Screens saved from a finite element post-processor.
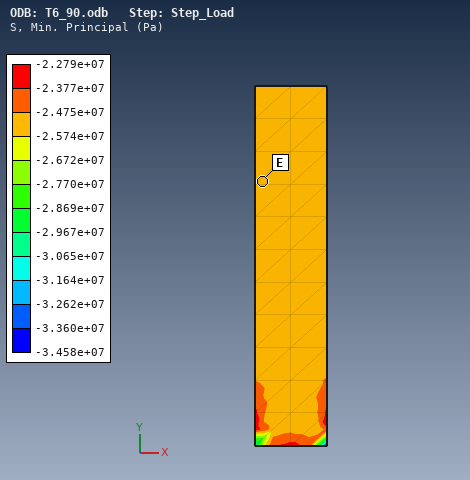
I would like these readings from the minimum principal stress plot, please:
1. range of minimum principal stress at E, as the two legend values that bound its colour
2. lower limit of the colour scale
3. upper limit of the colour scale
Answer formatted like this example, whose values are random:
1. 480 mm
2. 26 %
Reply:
1. -2.574e+07 to -2.475e+07 Pa
2. -3.458e+07 Pa
3. -2.279e+07 Pa
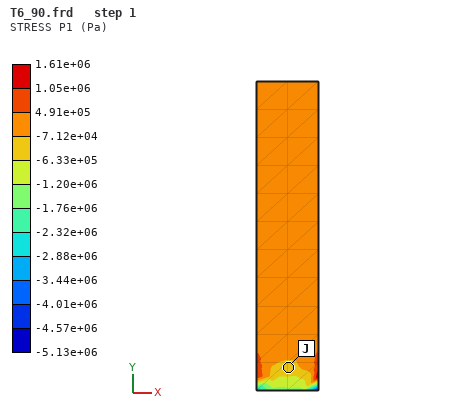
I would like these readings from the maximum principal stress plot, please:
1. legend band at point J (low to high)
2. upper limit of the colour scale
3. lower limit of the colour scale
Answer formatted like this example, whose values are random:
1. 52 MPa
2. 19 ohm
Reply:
1. -6.33e+05 to -7.12e+04 Pa
2. 1.61e+06 Pa
3. -5.13e+06 Pa
